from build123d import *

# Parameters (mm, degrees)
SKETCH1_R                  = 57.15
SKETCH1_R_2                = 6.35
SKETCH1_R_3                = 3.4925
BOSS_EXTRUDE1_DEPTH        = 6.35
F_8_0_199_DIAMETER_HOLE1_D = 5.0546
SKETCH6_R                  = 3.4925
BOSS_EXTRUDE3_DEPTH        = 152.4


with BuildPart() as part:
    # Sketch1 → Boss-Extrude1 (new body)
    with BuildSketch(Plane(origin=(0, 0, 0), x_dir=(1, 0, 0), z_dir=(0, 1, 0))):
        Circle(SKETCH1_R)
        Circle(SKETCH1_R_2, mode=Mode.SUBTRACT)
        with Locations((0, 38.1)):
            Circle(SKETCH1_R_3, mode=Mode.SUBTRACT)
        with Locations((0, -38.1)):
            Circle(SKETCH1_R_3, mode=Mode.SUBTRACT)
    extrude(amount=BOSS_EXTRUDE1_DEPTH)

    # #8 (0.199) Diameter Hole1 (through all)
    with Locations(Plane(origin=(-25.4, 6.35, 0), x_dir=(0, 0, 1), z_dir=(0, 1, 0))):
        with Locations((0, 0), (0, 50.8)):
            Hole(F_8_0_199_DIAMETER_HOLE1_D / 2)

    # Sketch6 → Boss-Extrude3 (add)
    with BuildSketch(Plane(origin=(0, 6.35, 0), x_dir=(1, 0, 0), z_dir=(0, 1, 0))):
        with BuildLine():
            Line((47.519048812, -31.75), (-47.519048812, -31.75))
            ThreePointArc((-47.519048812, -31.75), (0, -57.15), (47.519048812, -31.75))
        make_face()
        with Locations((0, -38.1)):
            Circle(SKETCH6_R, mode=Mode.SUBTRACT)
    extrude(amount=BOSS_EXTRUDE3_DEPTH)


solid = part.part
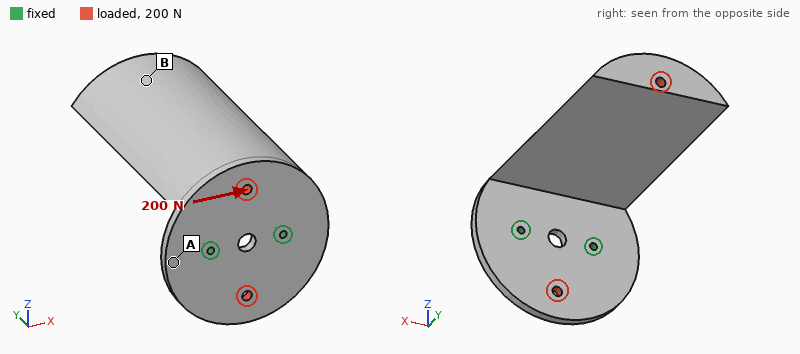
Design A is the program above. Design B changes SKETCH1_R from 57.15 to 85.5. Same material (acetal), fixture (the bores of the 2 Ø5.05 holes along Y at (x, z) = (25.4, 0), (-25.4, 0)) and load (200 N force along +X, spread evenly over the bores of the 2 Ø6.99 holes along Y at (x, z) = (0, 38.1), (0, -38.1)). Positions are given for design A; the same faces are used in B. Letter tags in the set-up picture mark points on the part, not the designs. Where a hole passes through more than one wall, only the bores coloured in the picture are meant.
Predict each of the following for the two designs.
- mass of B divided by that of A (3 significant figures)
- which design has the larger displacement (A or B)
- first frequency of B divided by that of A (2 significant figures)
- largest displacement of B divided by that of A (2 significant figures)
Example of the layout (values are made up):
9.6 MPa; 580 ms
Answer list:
1.25; A; 1.1; 0.79
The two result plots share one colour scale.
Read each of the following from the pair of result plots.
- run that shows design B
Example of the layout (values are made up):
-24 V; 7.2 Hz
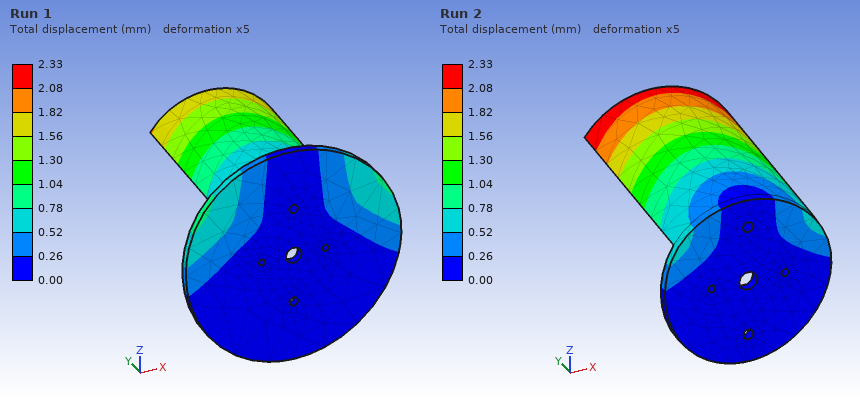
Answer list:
Run 1
